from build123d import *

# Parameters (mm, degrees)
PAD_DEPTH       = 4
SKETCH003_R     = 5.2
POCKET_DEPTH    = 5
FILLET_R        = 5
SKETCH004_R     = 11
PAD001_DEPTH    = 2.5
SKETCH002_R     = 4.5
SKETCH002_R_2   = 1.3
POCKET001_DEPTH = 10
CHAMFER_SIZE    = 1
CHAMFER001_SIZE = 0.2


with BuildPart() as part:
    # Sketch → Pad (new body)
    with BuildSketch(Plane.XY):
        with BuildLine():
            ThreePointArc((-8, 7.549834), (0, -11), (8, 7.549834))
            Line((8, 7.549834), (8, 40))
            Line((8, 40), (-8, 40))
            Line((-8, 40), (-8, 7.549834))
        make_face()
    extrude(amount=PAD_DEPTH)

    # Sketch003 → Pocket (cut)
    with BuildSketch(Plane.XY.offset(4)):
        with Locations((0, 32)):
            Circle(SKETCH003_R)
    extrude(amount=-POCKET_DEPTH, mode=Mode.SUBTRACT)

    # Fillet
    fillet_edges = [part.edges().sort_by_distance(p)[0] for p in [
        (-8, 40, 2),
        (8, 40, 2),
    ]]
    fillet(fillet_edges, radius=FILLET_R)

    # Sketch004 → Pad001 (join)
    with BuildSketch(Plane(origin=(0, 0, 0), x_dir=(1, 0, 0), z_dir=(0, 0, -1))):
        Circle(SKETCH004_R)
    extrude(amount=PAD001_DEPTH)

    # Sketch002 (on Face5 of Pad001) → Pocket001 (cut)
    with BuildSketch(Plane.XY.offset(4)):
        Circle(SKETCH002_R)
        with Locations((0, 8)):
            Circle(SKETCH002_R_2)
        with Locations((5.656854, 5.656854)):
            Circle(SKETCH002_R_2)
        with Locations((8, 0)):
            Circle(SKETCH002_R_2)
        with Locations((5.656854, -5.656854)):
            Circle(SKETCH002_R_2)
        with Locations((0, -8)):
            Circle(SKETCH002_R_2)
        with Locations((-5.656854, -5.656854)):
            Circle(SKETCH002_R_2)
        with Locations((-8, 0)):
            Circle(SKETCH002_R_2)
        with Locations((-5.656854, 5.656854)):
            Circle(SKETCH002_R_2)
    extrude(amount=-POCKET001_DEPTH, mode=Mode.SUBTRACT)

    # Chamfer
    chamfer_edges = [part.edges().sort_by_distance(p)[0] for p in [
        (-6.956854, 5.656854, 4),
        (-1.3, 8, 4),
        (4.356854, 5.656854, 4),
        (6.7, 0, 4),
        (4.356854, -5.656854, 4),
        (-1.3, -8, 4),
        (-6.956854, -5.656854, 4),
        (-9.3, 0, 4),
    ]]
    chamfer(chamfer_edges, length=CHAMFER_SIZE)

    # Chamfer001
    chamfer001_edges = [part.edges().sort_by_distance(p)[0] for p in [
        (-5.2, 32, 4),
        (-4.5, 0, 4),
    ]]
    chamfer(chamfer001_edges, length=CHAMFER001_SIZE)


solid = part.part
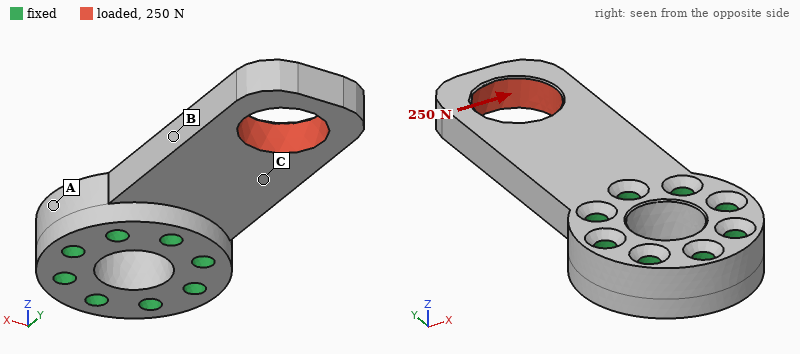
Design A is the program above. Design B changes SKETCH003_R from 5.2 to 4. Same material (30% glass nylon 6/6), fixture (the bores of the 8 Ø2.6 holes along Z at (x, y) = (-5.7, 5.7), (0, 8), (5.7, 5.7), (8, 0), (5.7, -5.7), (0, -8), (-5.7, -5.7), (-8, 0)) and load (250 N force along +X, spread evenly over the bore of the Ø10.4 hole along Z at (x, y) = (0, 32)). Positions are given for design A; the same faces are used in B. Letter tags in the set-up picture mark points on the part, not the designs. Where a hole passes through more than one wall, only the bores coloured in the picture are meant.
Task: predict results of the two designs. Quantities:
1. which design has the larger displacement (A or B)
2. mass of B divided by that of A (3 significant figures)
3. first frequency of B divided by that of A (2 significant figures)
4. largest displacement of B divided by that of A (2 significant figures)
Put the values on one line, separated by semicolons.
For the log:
A; 1.04; 0.93; 0.83
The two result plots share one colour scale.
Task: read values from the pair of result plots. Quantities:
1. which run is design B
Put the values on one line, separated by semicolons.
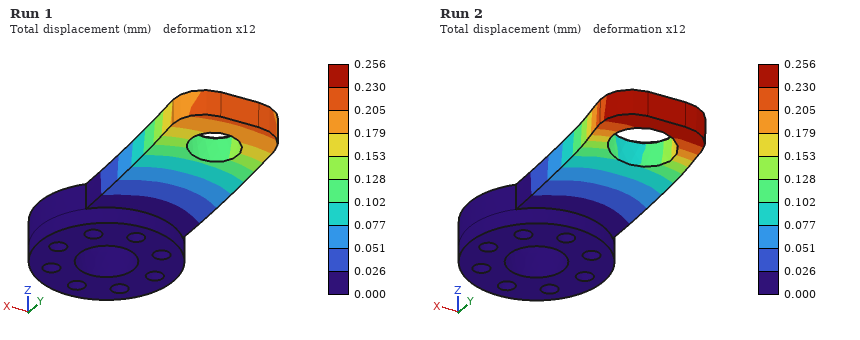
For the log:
Run 1
